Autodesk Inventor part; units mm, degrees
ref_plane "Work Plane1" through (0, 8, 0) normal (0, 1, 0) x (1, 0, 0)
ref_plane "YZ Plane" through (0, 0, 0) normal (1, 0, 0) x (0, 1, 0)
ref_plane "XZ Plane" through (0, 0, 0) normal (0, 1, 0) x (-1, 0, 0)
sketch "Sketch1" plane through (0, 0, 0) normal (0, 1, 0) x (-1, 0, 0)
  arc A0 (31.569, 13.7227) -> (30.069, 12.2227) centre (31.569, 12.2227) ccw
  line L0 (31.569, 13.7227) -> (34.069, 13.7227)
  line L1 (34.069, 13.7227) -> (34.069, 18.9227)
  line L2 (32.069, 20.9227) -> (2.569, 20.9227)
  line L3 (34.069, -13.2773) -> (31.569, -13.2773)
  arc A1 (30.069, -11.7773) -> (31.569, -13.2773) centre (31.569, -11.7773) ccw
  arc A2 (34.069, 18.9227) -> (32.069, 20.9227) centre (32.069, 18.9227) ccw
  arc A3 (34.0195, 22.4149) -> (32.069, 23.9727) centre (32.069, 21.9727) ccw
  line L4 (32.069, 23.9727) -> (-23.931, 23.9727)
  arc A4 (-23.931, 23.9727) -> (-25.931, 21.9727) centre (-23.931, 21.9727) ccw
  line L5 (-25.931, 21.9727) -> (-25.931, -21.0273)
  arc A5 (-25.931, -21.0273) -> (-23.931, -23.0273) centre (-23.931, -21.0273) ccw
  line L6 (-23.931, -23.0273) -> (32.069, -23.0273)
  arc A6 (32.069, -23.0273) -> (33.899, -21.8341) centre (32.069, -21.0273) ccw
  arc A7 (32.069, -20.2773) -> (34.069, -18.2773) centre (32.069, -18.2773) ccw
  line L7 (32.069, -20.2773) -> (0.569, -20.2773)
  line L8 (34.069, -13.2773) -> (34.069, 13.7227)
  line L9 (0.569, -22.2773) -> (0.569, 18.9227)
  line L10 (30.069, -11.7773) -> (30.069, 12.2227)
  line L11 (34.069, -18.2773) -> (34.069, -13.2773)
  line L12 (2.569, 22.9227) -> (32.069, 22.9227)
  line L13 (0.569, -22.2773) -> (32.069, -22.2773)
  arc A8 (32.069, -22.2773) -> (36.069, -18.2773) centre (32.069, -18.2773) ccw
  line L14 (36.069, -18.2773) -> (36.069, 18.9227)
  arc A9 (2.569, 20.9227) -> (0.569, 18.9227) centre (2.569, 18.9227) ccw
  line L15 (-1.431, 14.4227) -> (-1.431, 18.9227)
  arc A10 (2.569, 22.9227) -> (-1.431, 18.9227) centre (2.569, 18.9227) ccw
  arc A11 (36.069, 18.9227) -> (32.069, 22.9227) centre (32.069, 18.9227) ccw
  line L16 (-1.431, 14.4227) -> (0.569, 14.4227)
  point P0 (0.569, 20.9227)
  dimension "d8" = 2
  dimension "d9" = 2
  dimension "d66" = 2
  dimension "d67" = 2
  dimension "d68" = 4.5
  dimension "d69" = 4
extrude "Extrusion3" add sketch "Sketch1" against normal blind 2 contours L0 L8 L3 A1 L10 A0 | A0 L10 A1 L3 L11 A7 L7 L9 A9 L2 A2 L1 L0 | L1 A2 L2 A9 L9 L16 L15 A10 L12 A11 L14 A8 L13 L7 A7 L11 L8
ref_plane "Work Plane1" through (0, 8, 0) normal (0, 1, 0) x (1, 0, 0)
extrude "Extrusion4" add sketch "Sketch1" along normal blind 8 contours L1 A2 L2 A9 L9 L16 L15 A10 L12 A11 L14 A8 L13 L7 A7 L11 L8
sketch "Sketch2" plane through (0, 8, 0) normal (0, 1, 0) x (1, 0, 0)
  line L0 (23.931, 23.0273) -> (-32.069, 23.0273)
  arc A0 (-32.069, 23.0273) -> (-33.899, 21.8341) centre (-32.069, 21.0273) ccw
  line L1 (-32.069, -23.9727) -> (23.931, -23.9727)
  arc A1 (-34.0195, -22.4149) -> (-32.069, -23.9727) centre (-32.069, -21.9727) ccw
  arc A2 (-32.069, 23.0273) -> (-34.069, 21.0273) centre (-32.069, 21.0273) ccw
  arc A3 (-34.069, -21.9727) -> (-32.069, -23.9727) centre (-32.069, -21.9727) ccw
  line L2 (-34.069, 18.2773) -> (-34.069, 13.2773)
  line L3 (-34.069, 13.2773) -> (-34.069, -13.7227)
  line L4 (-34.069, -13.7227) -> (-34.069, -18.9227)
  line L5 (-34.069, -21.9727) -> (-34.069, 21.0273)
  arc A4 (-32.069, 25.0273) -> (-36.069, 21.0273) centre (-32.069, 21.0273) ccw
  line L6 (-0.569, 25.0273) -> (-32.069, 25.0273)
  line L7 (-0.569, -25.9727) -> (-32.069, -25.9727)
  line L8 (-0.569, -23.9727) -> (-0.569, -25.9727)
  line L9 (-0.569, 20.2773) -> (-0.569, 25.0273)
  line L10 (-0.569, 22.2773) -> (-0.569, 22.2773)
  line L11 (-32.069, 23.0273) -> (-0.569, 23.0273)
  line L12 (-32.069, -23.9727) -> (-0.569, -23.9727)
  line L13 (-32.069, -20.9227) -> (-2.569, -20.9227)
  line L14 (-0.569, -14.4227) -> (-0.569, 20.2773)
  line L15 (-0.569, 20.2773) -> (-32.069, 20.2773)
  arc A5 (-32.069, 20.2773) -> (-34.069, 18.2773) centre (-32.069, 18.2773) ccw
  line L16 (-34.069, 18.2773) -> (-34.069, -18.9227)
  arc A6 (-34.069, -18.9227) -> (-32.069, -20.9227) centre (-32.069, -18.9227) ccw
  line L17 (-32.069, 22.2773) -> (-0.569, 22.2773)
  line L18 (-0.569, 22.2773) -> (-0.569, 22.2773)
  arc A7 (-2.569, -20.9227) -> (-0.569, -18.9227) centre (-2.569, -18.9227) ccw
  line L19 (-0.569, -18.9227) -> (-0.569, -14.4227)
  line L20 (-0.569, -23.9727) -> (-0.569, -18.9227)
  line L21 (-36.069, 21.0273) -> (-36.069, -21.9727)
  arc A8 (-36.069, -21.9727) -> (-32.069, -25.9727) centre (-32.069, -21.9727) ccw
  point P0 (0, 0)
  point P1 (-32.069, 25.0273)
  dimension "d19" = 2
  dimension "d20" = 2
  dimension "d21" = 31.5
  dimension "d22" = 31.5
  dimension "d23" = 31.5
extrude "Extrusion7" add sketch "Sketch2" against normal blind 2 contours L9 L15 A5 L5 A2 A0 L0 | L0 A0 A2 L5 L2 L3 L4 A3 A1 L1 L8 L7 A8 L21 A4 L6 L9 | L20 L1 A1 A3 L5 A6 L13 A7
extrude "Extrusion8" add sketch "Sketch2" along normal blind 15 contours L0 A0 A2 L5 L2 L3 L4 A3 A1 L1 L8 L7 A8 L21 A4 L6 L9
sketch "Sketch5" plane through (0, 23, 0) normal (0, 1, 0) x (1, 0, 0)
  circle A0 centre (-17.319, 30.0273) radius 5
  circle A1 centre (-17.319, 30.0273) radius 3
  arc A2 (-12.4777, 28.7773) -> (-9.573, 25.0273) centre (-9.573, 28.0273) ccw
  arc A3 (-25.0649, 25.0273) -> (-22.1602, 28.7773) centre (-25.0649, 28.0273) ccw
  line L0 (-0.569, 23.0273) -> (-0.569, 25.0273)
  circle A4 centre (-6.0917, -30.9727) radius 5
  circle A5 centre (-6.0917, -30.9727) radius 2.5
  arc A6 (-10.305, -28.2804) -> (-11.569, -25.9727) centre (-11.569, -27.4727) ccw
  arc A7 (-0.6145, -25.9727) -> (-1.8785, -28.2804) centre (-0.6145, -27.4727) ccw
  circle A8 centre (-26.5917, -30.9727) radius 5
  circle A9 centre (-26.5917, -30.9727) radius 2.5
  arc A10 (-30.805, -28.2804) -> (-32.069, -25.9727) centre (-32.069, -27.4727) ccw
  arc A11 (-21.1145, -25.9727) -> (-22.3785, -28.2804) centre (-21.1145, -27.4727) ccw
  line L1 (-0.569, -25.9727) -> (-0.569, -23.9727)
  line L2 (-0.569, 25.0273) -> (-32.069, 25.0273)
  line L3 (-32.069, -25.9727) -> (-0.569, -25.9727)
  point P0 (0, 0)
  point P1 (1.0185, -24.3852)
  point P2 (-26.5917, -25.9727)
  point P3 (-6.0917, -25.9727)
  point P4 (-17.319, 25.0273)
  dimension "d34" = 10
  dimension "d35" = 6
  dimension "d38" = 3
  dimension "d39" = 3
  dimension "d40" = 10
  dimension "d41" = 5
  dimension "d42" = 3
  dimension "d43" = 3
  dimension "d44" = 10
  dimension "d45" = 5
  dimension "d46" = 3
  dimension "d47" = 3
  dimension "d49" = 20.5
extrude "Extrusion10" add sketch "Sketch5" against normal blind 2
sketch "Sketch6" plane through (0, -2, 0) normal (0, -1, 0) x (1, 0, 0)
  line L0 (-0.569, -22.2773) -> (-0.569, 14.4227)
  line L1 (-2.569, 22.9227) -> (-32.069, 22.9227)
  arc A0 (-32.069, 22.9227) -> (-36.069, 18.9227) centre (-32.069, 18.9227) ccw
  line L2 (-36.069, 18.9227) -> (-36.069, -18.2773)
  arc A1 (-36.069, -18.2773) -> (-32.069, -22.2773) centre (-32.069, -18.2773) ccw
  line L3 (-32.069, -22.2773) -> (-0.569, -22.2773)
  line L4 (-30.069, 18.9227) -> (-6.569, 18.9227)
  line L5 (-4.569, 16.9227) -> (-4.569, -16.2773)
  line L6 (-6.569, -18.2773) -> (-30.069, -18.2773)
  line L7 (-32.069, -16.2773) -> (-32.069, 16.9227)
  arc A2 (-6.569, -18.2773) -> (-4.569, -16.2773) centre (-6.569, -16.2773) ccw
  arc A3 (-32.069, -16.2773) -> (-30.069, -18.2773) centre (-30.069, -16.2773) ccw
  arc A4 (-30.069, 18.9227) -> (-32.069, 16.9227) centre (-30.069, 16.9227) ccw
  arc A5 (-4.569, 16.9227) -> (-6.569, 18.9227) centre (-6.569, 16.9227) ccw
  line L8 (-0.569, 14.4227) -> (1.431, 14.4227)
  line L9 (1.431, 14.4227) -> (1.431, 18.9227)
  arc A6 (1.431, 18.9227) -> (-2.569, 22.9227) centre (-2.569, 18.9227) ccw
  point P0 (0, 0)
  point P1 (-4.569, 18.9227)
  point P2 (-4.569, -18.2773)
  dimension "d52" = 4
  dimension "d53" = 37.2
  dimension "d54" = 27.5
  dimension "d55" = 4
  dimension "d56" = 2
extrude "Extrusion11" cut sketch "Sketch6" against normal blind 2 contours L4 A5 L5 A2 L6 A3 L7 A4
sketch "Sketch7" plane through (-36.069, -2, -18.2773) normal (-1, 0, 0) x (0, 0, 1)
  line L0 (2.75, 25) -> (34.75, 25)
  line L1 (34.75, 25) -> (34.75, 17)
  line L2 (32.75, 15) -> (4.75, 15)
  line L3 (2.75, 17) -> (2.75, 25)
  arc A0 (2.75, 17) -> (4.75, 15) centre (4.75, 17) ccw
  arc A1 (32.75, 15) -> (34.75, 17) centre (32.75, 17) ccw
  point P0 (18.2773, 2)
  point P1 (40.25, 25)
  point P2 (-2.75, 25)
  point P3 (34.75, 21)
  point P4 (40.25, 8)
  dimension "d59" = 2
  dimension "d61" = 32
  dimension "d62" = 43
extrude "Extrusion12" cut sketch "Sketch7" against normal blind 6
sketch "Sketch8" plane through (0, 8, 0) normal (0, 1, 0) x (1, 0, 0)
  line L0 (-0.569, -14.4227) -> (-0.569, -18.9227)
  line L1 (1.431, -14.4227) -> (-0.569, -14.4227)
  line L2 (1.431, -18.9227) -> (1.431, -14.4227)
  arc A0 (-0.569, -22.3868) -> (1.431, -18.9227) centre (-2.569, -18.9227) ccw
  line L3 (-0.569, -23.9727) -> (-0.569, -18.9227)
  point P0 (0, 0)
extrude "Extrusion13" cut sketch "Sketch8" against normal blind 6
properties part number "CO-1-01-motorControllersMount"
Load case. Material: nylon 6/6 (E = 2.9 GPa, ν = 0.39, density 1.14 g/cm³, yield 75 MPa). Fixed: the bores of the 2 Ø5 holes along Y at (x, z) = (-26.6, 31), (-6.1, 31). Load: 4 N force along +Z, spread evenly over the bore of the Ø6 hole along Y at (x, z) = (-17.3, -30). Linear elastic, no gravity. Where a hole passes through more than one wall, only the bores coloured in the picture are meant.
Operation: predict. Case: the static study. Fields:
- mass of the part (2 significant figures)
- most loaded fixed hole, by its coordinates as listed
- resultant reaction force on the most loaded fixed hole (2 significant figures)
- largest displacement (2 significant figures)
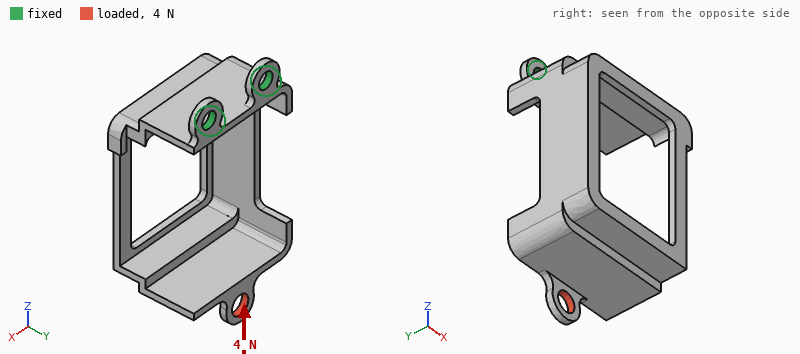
7.5 g
(-6.1, 31)
2.3 N
0.97 mm
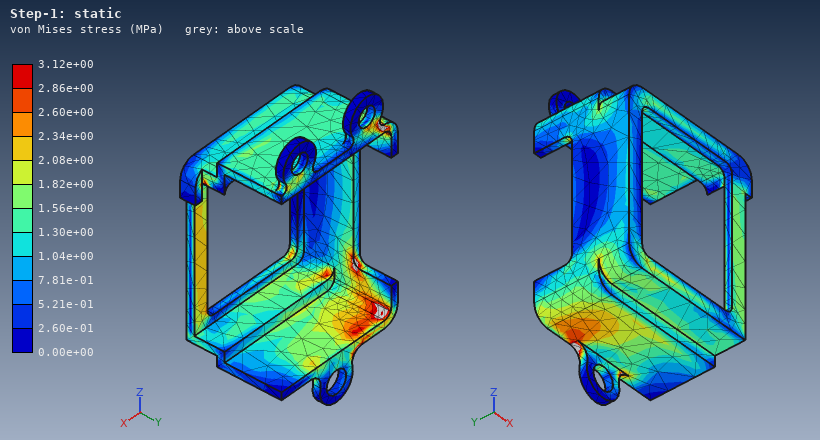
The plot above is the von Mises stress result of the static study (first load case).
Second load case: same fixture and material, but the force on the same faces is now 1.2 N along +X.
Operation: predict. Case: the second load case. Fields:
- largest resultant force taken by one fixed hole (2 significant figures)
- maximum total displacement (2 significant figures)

2.4 N
0.88 mm
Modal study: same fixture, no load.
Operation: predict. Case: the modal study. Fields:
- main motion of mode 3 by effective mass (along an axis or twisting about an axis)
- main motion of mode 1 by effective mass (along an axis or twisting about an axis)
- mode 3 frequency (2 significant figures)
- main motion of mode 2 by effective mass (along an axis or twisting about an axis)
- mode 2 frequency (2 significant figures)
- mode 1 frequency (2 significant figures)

along Z
along Y
350 Hz
along X
140 Hz
97 Hz
